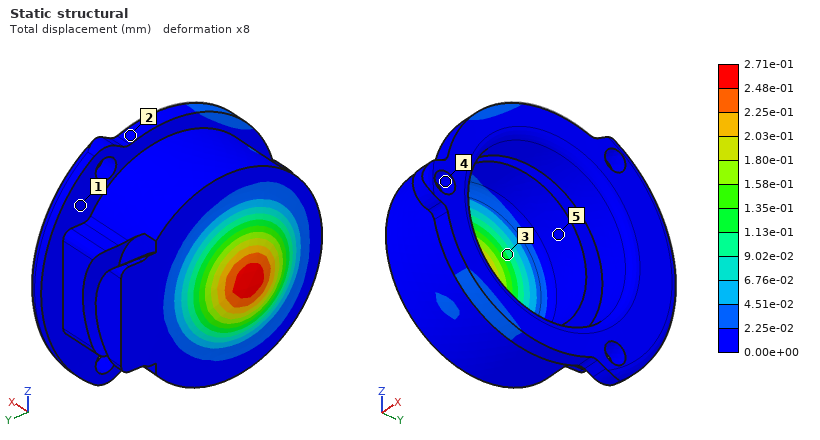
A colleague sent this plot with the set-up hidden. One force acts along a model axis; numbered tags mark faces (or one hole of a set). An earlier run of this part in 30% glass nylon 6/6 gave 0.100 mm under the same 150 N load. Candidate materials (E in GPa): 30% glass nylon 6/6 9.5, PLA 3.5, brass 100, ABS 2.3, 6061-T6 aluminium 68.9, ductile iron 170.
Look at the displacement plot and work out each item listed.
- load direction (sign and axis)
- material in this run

-X
PLA
